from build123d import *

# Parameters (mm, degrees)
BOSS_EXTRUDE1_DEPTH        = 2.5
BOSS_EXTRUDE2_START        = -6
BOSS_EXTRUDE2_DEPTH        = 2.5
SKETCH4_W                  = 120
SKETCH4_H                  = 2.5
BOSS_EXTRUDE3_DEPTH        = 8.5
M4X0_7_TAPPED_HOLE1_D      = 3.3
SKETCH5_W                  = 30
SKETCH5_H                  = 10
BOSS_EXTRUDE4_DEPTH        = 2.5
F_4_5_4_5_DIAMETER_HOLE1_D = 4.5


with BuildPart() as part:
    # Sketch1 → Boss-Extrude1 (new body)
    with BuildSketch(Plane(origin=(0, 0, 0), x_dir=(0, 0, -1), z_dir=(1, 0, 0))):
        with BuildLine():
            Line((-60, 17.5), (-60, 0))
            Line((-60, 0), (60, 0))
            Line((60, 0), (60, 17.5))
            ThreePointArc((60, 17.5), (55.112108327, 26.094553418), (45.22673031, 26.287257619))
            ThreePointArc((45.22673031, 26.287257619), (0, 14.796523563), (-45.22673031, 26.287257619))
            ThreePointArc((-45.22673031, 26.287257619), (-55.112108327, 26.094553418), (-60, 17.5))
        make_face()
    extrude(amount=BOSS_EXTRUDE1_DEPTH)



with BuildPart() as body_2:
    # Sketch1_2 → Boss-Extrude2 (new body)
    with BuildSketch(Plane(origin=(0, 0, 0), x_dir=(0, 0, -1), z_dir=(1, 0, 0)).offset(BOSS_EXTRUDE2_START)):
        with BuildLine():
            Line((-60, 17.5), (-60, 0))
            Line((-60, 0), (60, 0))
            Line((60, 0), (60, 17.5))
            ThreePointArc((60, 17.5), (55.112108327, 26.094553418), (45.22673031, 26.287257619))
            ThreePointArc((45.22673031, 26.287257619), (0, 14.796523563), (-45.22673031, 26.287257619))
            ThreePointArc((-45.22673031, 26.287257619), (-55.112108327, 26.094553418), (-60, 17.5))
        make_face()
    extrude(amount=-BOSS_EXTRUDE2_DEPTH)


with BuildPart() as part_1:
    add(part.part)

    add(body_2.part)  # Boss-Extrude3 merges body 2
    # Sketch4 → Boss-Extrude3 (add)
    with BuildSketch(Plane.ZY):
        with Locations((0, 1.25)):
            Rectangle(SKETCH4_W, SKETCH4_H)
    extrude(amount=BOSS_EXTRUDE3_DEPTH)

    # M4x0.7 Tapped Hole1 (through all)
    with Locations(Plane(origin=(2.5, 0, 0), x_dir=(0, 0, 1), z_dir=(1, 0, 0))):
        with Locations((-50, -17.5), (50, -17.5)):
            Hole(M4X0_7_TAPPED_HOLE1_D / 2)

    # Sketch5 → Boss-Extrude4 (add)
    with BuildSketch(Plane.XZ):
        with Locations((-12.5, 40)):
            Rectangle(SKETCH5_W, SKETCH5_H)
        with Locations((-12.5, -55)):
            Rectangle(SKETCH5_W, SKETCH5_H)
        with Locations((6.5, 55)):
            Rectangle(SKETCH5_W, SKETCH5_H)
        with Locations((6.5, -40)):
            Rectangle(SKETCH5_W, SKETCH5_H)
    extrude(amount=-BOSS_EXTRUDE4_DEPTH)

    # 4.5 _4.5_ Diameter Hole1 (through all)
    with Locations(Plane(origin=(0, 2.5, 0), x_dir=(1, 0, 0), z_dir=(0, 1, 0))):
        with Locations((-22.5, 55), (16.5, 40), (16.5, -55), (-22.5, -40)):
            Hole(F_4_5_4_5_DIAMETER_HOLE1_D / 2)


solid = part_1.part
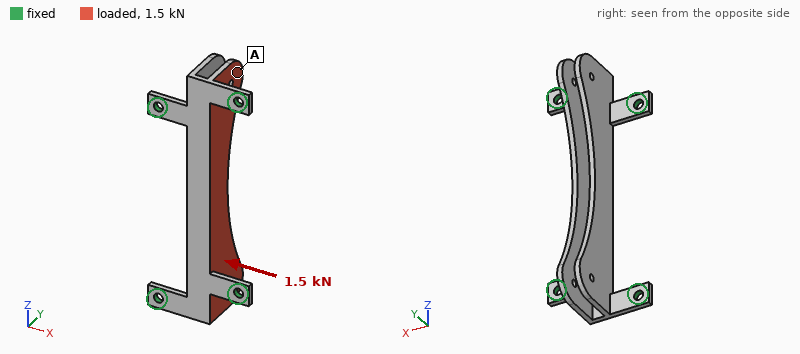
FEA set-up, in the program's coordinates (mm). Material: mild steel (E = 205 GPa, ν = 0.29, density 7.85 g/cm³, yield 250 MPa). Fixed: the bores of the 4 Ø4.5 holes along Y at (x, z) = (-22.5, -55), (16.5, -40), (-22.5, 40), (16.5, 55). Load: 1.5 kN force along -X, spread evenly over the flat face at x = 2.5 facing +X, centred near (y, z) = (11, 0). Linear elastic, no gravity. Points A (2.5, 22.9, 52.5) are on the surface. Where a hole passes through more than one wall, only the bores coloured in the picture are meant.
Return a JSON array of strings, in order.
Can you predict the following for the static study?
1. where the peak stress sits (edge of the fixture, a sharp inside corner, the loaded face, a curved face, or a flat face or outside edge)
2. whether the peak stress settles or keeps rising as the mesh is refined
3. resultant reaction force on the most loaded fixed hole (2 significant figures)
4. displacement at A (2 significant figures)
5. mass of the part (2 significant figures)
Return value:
["edge of the fixture", "keeps rising", "780 N", "0.13 mm", "120 g"]
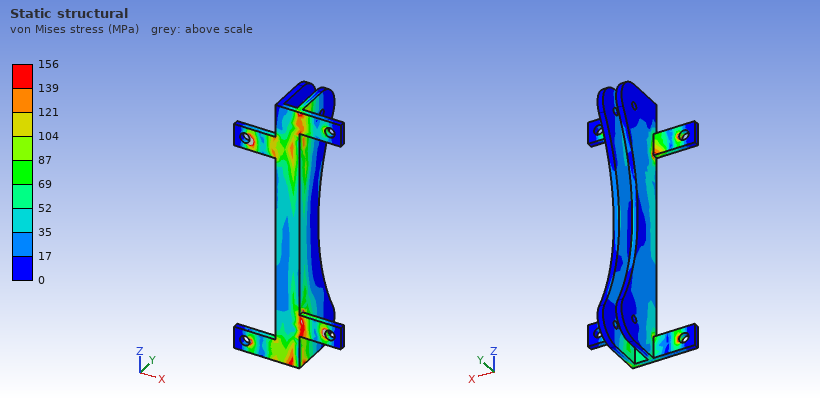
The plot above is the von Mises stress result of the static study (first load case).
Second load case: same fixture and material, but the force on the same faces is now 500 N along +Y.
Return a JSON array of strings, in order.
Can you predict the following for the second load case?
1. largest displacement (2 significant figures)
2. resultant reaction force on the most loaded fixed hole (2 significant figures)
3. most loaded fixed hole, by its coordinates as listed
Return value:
["30 µm", "210 N", "(16.5, -40)"]
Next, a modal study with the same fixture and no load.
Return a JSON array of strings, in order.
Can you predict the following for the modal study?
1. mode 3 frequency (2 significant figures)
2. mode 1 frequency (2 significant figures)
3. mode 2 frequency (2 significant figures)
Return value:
["3000 Hz", "2400 Hz", "2500 Hz"]
